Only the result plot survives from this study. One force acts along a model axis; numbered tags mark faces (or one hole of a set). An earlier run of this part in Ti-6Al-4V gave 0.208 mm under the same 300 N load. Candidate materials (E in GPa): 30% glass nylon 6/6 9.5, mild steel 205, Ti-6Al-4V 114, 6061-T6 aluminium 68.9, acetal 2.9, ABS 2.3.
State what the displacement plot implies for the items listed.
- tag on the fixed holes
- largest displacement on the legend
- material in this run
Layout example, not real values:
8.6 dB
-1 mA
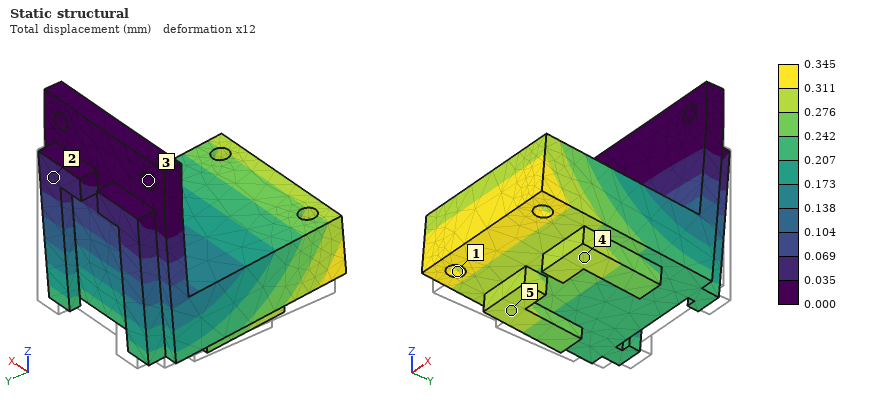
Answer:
3
0.345 mm
6061-T6 aluminium
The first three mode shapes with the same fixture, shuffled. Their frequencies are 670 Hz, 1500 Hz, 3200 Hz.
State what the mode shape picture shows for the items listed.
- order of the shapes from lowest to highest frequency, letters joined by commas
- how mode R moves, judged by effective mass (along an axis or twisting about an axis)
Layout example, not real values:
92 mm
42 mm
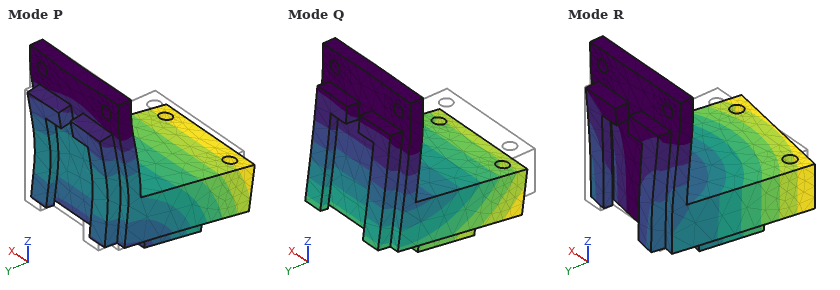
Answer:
Q, R, P
along X
